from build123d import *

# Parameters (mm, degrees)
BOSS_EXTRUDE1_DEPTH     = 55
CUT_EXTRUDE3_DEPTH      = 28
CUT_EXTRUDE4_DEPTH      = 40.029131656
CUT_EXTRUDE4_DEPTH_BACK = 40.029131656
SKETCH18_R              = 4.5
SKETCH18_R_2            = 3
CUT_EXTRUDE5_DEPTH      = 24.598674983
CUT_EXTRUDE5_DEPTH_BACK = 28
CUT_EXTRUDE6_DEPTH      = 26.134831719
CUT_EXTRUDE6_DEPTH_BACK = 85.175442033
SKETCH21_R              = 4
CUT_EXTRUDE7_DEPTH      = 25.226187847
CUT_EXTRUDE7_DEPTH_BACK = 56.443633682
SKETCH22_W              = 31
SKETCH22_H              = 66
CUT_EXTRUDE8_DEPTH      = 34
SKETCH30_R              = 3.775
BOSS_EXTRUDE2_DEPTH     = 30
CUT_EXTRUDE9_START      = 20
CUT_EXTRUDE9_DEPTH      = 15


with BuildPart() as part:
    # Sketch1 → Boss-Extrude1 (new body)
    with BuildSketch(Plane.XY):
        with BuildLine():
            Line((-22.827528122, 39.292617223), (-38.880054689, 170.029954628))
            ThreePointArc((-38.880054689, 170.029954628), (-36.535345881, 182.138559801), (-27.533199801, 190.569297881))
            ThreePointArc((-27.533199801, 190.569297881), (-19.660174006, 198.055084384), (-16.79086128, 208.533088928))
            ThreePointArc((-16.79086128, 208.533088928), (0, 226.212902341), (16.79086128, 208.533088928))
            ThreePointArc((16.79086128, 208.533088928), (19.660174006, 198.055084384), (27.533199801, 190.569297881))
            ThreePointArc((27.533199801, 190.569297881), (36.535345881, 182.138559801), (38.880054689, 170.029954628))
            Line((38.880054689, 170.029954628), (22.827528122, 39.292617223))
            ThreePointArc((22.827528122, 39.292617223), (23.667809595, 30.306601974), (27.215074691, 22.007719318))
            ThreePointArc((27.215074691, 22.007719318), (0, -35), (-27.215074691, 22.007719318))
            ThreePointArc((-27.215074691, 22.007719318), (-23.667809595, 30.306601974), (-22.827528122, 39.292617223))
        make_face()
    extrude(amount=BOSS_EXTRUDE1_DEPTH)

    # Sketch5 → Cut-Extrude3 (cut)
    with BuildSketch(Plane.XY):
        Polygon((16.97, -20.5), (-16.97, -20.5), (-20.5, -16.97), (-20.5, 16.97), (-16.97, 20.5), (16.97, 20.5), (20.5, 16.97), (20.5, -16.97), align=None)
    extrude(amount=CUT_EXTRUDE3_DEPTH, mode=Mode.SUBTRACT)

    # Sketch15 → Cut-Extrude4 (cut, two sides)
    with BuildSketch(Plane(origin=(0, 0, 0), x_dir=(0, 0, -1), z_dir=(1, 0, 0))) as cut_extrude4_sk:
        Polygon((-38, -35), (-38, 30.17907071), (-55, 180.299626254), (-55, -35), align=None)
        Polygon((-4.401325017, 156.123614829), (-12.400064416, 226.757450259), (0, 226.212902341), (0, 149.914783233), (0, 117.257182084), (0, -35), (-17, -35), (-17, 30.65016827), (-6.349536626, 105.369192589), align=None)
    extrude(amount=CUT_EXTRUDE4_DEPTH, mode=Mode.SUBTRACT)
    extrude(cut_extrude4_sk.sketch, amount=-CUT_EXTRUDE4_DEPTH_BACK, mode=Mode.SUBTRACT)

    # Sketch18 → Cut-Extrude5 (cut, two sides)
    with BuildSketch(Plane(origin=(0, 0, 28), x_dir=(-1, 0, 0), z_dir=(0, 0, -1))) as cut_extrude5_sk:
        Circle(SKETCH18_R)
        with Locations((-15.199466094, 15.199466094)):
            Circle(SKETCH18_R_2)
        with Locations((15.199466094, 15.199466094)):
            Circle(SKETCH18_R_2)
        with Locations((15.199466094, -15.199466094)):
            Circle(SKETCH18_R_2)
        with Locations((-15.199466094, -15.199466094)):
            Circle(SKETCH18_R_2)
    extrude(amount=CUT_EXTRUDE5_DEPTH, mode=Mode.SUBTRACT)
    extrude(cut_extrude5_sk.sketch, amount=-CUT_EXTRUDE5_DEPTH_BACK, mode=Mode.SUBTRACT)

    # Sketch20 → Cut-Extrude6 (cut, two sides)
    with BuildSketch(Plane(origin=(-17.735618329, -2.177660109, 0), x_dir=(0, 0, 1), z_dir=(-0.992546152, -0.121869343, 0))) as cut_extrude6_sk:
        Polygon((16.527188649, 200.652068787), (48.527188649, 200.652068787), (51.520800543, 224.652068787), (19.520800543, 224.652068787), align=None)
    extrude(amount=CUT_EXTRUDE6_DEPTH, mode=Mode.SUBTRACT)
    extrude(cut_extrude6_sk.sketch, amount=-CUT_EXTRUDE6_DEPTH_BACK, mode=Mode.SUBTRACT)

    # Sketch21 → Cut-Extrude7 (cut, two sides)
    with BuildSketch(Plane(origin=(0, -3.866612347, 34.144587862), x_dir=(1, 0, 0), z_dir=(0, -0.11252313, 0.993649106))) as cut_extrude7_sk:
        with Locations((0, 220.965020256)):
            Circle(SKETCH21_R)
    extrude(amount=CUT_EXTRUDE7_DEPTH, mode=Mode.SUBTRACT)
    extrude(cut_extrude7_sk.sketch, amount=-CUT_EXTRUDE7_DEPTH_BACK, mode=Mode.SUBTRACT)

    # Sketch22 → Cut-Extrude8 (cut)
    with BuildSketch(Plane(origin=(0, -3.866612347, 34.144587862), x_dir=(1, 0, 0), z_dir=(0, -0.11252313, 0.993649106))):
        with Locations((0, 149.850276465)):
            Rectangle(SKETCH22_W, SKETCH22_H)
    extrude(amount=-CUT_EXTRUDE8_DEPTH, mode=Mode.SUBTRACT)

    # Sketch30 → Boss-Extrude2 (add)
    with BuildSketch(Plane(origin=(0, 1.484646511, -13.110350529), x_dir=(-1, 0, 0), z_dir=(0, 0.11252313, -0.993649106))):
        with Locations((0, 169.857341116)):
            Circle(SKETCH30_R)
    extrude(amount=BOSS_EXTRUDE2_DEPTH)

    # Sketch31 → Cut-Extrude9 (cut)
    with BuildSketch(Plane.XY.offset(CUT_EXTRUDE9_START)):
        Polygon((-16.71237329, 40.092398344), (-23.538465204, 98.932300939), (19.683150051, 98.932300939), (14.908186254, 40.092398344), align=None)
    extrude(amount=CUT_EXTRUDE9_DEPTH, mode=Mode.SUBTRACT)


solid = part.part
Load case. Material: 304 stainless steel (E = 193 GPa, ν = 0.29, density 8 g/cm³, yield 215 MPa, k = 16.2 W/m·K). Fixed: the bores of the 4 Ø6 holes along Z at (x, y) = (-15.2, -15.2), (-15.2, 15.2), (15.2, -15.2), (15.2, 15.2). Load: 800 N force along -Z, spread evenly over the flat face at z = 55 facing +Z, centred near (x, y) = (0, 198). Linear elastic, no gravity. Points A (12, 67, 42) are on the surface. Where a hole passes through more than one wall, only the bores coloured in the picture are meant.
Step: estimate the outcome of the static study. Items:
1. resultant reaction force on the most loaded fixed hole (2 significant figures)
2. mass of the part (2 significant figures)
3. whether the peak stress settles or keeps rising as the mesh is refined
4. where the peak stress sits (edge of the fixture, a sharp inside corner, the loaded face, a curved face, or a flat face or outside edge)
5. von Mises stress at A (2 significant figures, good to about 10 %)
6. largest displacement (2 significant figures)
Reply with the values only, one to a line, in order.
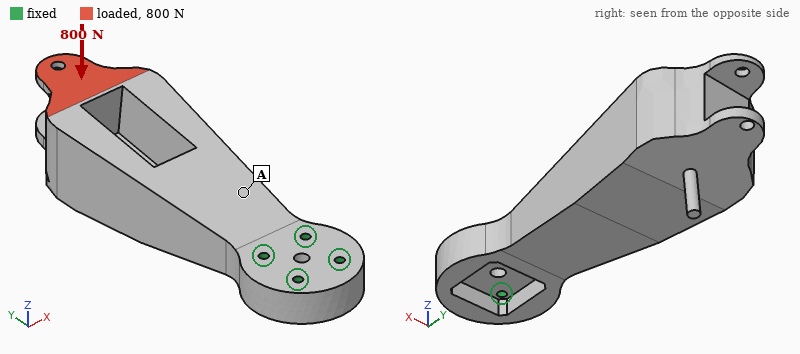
2.2 kN
3.1 kg
keeps rising
edge of the fixture
15 MPa
0.28 mm
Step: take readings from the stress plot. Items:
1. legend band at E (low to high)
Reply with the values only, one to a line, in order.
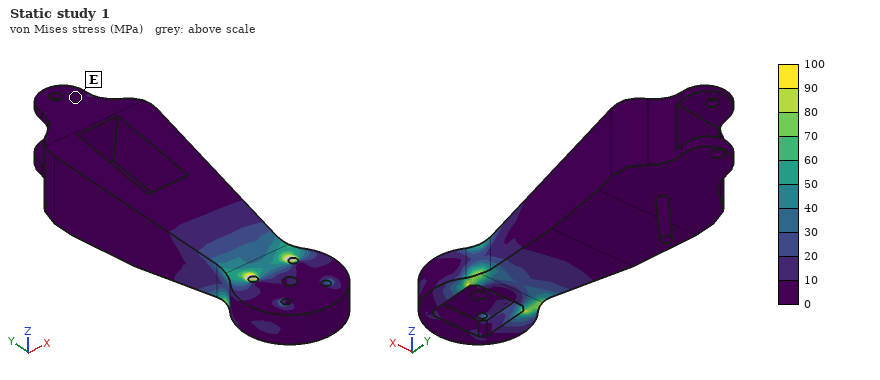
0 to 10 MPa
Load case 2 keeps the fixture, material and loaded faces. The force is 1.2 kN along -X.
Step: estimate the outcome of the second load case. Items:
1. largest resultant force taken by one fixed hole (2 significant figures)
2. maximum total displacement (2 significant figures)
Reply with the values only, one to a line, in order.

4.7 kN
92 µm
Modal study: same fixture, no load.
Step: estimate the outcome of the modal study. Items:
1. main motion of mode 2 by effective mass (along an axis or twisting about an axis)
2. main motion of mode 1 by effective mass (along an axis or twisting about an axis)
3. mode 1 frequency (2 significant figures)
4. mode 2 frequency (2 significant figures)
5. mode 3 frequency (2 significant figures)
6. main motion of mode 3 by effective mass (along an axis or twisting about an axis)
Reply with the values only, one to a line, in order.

along X
along Z
270 Hz
620 Hz
1500 Hz
twisting about Y
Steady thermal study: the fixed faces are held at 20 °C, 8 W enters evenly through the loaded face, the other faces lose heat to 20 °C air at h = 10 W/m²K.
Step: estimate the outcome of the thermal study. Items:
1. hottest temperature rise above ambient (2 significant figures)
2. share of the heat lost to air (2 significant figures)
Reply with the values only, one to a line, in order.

40 K
83 %
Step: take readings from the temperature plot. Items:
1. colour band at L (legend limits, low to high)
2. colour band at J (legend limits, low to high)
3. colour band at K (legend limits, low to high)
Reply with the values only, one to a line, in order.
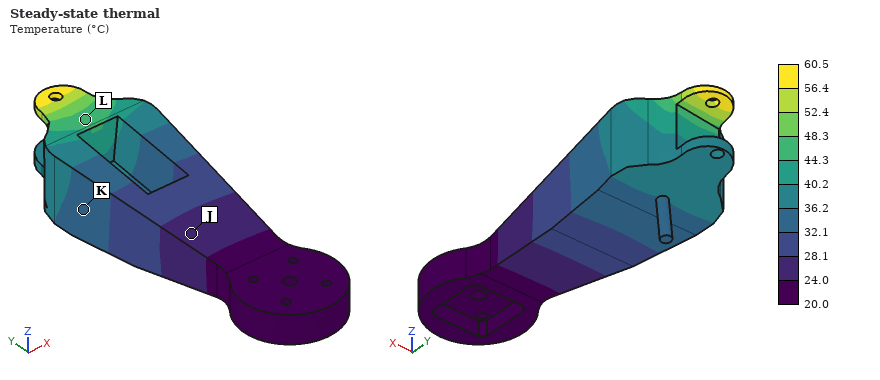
44.3 to 48.3 °C
24.0 to 28.1 °C
32.1 to 36.2 °C
